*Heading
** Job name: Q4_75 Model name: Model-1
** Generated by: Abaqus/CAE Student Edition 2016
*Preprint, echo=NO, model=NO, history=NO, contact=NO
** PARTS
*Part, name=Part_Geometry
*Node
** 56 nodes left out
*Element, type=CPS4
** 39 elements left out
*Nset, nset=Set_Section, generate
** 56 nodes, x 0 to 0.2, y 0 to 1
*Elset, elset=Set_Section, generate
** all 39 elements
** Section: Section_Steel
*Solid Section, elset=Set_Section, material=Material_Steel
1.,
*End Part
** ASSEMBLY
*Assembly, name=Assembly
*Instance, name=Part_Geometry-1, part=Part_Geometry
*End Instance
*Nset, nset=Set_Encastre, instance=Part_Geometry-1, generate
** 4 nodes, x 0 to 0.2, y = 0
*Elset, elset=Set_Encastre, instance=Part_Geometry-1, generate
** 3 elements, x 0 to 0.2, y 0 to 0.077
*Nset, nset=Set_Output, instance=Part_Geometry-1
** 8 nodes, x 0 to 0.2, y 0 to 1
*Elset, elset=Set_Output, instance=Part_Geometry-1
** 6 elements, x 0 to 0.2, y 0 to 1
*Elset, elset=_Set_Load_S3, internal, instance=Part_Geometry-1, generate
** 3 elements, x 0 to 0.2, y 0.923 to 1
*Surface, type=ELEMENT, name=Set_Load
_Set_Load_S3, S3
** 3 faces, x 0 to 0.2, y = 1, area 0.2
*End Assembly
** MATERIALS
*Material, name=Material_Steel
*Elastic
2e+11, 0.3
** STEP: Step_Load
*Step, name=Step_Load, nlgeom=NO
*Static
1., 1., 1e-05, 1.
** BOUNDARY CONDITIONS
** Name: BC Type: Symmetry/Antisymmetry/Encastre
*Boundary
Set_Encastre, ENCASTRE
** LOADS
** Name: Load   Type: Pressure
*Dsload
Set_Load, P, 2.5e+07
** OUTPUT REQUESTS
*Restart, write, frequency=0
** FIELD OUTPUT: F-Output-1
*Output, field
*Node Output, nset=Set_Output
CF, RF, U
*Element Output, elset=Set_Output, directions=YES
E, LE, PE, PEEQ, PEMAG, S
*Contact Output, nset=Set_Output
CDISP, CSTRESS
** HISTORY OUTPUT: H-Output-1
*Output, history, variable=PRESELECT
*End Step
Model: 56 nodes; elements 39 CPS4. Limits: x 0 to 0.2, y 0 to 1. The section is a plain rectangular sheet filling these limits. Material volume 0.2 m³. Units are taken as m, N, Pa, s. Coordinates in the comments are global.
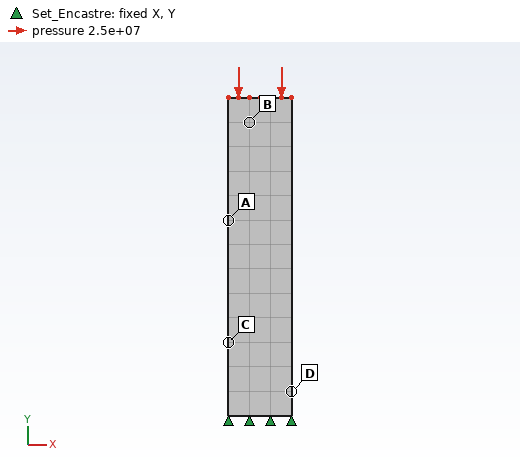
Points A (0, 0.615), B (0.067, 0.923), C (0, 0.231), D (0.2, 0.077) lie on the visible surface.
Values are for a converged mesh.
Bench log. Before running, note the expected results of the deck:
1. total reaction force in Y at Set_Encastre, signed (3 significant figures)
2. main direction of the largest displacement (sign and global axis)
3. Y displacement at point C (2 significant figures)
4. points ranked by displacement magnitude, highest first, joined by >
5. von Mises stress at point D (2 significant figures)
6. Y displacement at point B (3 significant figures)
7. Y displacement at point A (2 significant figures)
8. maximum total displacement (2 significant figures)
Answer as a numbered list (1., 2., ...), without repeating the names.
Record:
1. 5.00e+06 N
2. -Y
3. -2.8e-05 m
4. B > A > C > D
5. 2.5e+07 Pa
6. -1.15e-04 m
7. -7.7e-05 m
8. 1.2e-04 m
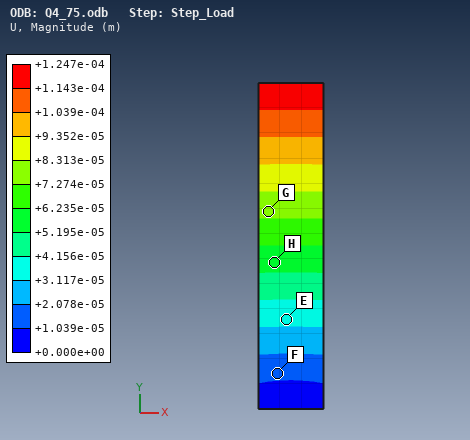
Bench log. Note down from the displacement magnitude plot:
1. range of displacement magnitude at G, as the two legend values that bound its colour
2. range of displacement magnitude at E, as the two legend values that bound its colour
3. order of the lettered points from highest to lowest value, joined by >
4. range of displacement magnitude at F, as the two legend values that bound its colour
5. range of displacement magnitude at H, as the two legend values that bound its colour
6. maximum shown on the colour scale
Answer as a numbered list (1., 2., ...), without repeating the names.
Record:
1. +7.274e-05 to +8.313e-05 m
2. +3.117e-05 to +4.156e-05 m
3. G > H > E > F
4. +1.039e-05 to +2.078e-05 m
5. +5.195e-05 to +6.235e-05 m
6. +1.247e-04 m
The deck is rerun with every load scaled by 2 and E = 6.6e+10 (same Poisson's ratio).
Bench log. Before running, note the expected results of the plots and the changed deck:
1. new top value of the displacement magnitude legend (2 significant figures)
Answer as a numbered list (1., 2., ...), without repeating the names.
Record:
1. 7.6e-04 m
